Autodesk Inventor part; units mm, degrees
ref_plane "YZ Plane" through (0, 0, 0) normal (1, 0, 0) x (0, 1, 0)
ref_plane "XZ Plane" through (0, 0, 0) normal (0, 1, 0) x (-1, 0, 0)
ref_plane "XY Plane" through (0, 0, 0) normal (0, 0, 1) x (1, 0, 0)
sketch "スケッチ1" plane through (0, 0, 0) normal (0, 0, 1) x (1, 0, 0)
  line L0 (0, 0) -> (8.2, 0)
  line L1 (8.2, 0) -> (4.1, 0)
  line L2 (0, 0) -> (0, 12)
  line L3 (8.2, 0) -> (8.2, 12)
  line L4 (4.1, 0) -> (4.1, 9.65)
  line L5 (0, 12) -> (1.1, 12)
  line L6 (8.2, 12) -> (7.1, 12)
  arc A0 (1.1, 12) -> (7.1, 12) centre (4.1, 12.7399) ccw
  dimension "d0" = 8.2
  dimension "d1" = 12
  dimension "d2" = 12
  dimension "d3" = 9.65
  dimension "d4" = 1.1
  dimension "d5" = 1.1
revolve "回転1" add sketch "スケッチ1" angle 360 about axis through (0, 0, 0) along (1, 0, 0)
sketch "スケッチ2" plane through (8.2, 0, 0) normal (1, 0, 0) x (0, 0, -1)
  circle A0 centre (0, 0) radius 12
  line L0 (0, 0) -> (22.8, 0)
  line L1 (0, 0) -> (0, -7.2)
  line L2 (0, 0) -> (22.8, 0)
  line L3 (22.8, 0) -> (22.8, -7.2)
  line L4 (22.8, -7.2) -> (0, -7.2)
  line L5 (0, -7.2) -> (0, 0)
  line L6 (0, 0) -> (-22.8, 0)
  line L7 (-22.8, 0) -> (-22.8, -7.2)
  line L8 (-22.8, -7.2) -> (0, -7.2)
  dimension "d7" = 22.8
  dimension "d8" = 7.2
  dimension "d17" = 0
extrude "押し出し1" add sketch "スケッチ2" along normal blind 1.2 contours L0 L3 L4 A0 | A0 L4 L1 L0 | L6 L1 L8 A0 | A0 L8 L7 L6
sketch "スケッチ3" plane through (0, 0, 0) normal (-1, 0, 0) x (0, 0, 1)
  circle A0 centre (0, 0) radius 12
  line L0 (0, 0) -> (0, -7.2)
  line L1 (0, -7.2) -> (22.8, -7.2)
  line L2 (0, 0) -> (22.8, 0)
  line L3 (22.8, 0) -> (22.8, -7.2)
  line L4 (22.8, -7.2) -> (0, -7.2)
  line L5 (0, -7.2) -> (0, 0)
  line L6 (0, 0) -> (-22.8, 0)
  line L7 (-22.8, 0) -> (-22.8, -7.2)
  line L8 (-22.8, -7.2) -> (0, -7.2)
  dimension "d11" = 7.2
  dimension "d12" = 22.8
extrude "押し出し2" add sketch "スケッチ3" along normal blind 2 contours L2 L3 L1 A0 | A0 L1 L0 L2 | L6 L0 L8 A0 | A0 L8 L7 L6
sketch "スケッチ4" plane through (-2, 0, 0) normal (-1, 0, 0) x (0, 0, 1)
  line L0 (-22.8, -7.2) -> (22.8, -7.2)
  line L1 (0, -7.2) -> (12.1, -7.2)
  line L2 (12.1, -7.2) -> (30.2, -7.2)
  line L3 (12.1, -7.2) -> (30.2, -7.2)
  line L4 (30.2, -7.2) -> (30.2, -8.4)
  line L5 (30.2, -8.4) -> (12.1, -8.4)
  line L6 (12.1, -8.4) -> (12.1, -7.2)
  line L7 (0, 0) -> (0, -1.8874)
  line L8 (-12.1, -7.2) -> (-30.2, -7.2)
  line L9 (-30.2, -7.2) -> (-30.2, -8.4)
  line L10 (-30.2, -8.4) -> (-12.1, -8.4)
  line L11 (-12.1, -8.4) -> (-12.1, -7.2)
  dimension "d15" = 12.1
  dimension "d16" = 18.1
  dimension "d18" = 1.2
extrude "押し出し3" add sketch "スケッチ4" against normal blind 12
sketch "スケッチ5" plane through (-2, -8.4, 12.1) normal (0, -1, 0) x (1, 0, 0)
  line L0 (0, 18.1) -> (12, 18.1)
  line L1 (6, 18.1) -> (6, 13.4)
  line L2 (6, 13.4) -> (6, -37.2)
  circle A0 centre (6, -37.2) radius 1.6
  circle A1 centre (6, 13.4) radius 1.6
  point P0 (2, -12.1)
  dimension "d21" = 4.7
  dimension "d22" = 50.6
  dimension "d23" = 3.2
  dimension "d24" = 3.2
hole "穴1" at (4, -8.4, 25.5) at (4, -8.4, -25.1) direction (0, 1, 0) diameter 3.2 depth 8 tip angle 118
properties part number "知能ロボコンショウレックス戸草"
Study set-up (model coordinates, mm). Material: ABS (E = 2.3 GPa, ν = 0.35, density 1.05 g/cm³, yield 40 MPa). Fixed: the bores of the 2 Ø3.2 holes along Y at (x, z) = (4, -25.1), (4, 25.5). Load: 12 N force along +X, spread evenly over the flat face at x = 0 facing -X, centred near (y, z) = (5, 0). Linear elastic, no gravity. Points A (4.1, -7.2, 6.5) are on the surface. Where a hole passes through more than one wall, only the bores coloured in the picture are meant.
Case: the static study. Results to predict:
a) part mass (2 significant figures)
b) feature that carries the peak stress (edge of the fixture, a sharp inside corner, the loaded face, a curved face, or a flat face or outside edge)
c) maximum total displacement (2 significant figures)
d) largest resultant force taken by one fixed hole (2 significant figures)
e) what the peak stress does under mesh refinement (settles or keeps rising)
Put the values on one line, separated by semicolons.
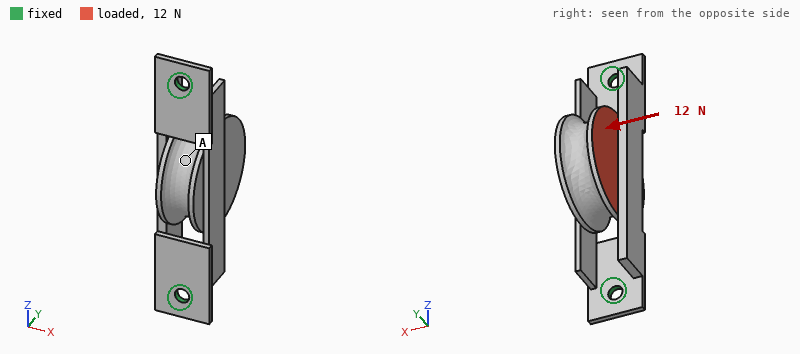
4.8 g; edge of the fixture; 0.65 mm; 6.6 N; keeps rising
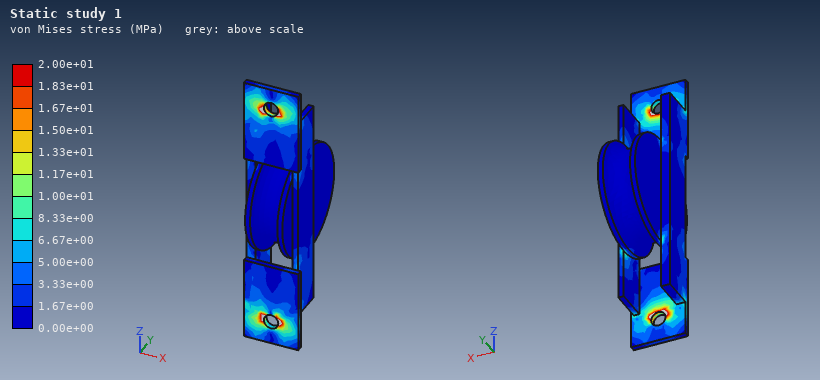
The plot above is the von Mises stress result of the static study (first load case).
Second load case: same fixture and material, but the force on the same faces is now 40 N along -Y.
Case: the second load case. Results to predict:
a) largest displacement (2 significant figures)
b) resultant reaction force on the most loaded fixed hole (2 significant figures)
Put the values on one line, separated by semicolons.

0.62 mm; 34 N
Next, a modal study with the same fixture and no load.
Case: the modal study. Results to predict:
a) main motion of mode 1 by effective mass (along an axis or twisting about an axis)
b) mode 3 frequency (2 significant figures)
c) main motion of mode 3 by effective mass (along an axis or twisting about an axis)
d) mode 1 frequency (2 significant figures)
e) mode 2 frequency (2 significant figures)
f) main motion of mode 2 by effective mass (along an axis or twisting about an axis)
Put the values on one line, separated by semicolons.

along X; 2500 Hz; along X; 570 Hz; 1400 Hz; along Y
